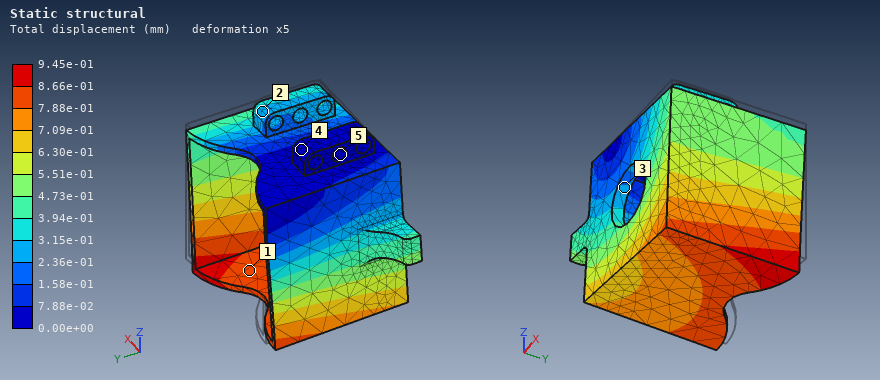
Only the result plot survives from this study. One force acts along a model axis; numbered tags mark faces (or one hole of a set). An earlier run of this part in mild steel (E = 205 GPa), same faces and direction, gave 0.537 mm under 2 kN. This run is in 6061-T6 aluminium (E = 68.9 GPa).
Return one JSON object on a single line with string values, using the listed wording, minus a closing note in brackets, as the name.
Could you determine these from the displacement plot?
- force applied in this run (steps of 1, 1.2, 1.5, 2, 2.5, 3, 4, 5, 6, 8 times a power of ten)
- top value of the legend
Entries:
{"force applied in this run": "1.2 kN", "top value of the legend": "9.45e-01 mm"}
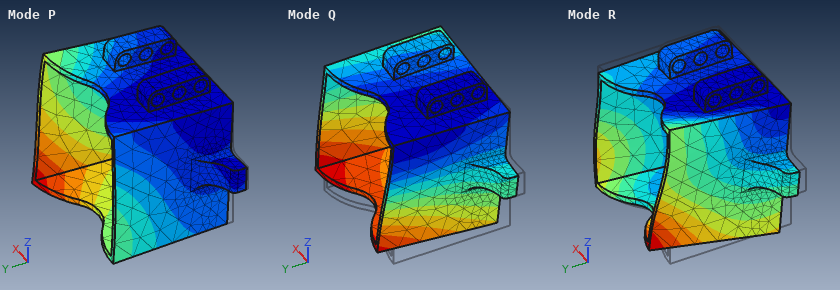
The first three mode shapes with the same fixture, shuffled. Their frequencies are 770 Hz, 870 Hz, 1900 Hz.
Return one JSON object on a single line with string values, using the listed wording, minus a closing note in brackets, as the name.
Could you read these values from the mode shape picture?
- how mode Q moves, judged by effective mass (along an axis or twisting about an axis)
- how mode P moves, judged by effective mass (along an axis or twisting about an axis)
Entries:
{"how mode Q moves, judged by effective mass": "along X", "how mode P moves, judged by effective mass": "along Y"}
